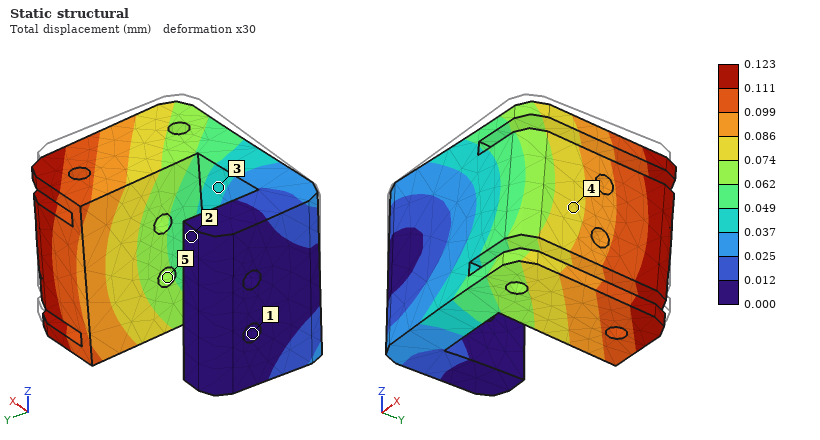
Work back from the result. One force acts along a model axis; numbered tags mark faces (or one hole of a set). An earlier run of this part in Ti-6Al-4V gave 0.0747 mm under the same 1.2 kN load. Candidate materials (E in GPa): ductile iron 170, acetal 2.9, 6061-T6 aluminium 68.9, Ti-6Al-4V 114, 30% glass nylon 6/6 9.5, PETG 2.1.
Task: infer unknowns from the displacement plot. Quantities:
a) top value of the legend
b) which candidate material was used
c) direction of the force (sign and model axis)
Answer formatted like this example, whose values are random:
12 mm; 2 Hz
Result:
0.123 mm; 6061-T6 aluminium; -Z
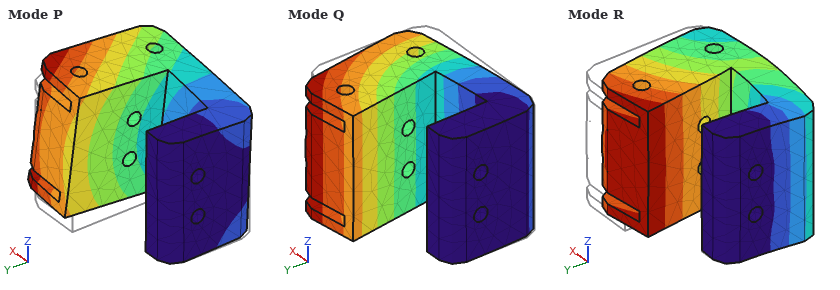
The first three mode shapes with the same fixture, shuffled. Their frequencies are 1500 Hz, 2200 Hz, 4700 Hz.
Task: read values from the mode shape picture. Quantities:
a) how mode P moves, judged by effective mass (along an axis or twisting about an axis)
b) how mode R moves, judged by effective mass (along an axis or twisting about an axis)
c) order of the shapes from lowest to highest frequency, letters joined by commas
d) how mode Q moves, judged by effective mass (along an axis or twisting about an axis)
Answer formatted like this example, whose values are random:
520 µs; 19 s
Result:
along Z; along X; Q, P, R; along Y
